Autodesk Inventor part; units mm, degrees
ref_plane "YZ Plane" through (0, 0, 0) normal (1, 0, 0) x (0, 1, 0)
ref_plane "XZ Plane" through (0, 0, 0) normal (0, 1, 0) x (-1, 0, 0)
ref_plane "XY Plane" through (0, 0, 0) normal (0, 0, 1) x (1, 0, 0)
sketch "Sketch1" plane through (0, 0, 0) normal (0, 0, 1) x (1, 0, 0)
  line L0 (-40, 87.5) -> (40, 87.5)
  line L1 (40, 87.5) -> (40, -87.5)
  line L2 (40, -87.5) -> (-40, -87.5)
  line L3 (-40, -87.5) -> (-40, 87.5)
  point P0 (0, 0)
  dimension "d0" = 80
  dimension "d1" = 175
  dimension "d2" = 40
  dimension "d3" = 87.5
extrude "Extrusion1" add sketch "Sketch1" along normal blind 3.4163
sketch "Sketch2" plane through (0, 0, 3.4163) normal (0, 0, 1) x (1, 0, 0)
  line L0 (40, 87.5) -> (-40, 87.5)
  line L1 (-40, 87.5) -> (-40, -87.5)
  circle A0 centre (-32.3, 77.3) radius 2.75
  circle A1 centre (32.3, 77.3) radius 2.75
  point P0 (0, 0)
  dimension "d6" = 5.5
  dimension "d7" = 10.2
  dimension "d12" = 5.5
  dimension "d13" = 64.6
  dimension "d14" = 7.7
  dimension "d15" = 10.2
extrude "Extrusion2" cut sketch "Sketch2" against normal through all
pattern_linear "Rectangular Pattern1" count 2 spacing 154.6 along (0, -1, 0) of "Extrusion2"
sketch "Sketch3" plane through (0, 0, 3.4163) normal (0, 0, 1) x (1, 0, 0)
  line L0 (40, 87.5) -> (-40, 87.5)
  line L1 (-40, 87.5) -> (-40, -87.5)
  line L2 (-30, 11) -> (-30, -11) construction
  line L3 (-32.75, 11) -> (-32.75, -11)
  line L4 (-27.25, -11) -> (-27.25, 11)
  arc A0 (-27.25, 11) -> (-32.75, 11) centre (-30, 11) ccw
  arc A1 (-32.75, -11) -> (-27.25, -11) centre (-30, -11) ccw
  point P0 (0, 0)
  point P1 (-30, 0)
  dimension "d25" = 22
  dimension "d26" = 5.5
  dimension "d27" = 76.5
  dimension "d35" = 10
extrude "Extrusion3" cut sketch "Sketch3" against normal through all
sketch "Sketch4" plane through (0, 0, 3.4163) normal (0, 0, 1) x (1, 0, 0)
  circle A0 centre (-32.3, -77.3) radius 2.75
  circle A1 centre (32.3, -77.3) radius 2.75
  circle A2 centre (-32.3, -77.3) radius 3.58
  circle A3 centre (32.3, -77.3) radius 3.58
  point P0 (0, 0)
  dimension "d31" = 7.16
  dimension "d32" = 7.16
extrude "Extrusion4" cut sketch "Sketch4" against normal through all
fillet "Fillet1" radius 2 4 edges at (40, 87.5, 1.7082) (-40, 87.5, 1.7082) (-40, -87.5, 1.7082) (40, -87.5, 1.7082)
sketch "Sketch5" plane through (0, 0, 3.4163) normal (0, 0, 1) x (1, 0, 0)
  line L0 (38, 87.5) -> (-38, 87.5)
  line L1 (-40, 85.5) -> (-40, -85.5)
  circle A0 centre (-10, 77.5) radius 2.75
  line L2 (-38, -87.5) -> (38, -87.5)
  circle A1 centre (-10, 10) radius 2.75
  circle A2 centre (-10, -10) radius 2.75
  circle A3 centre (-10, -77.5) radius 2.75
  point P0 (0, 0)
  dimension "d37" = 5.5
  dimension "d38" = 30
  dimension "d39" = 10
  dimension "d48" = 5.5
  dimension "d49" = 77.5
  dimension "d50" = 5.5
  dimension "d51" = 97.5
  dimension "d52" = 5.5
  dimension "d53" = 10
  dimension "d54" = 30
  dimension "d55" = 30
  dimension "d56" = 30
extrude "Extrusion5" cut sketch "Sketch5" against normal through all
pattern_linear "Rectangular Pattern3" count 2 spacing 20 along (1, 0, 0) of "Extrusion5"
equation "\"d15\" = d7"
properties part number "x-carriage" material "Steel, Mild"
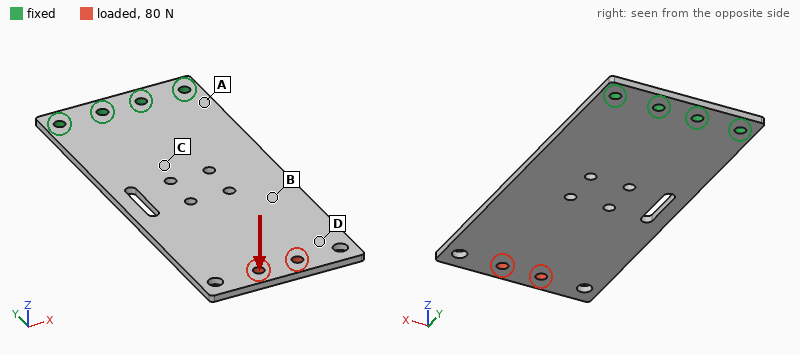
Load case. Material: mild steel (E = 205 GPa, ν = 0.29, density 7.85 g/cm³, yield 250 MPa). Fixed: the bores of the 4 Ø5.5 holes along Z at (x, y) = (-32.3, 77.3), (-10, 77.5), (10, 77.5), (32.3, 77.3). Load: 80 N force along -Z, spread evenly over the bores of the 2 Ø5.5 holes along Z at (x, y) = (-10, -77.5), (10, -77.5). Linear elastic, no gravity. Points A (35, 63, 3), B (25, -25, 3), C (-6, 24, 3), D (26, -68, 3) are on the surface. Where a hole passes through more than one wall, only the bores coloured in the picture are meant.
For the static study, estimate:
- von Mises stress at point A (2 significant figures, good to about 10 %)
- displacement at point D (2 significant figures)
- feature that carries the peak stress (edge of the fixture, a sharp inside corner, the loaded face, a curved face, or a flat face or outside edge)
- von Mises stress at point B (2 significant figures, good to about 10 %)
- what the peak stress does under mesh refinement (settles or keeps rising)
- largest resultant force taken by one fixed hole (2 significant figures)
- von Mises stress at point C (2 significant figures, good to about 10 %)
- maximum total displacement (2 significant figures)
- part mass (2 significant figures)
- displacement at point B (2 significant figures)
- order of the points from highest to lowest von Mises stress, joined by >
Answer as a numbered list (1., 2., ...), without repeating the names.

1. 71 MPa
2. 1.6 mm
3. edge of the fixture
4. 29 MPa
5. keeps rising
6. 63 N
7. 48 MPa
8. 2.0 mm
9. 360 g
10. 0.89 mm
11. A > C > B > D
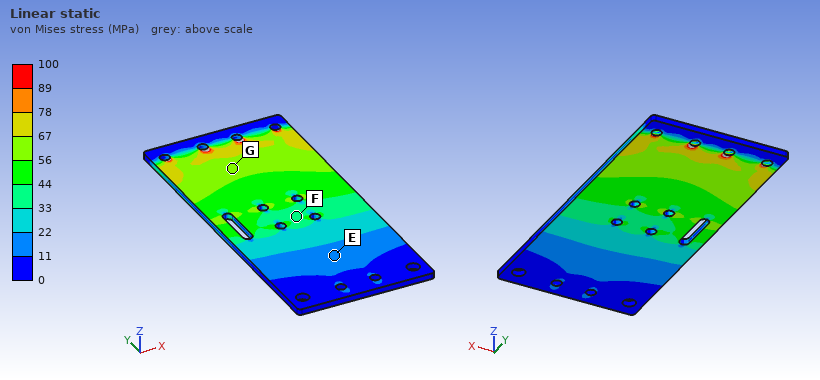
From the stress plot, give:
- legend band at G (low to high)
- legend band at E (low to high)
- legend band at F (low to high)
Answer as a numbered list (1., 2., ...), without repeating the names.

1. 56 to 67 MPa
2. 11 to 22 MPa
3. 33 to 44 MPa
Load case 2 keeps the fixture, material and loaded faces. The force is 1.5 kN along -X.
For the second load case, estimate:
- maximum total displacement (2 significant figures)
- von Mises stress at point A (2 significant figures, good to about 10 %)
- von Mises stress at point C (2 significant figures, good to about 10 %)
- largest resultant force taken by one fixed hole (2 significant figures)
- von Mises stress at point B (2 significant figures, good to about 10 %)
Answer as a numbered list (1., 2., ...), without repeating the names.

1. 89 µm
2. 54 MPa
3. 16 MPa
4. 3.2 kN
5. 16 MPa
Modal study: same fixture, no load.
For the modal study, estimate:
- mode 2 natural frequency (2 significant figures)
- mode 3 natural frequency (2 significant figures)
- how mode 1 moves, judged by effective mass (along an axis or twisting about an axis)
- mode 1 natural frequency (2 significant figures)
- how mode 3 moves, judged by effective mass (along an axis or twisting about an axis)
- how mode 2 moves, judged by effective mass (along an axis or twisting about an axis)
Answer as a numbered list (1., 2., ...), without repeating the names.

1. 470 Hz
2. 670 Hz
3. along Z
4. 110 Hz
5. along Z
6. twisting about Y
